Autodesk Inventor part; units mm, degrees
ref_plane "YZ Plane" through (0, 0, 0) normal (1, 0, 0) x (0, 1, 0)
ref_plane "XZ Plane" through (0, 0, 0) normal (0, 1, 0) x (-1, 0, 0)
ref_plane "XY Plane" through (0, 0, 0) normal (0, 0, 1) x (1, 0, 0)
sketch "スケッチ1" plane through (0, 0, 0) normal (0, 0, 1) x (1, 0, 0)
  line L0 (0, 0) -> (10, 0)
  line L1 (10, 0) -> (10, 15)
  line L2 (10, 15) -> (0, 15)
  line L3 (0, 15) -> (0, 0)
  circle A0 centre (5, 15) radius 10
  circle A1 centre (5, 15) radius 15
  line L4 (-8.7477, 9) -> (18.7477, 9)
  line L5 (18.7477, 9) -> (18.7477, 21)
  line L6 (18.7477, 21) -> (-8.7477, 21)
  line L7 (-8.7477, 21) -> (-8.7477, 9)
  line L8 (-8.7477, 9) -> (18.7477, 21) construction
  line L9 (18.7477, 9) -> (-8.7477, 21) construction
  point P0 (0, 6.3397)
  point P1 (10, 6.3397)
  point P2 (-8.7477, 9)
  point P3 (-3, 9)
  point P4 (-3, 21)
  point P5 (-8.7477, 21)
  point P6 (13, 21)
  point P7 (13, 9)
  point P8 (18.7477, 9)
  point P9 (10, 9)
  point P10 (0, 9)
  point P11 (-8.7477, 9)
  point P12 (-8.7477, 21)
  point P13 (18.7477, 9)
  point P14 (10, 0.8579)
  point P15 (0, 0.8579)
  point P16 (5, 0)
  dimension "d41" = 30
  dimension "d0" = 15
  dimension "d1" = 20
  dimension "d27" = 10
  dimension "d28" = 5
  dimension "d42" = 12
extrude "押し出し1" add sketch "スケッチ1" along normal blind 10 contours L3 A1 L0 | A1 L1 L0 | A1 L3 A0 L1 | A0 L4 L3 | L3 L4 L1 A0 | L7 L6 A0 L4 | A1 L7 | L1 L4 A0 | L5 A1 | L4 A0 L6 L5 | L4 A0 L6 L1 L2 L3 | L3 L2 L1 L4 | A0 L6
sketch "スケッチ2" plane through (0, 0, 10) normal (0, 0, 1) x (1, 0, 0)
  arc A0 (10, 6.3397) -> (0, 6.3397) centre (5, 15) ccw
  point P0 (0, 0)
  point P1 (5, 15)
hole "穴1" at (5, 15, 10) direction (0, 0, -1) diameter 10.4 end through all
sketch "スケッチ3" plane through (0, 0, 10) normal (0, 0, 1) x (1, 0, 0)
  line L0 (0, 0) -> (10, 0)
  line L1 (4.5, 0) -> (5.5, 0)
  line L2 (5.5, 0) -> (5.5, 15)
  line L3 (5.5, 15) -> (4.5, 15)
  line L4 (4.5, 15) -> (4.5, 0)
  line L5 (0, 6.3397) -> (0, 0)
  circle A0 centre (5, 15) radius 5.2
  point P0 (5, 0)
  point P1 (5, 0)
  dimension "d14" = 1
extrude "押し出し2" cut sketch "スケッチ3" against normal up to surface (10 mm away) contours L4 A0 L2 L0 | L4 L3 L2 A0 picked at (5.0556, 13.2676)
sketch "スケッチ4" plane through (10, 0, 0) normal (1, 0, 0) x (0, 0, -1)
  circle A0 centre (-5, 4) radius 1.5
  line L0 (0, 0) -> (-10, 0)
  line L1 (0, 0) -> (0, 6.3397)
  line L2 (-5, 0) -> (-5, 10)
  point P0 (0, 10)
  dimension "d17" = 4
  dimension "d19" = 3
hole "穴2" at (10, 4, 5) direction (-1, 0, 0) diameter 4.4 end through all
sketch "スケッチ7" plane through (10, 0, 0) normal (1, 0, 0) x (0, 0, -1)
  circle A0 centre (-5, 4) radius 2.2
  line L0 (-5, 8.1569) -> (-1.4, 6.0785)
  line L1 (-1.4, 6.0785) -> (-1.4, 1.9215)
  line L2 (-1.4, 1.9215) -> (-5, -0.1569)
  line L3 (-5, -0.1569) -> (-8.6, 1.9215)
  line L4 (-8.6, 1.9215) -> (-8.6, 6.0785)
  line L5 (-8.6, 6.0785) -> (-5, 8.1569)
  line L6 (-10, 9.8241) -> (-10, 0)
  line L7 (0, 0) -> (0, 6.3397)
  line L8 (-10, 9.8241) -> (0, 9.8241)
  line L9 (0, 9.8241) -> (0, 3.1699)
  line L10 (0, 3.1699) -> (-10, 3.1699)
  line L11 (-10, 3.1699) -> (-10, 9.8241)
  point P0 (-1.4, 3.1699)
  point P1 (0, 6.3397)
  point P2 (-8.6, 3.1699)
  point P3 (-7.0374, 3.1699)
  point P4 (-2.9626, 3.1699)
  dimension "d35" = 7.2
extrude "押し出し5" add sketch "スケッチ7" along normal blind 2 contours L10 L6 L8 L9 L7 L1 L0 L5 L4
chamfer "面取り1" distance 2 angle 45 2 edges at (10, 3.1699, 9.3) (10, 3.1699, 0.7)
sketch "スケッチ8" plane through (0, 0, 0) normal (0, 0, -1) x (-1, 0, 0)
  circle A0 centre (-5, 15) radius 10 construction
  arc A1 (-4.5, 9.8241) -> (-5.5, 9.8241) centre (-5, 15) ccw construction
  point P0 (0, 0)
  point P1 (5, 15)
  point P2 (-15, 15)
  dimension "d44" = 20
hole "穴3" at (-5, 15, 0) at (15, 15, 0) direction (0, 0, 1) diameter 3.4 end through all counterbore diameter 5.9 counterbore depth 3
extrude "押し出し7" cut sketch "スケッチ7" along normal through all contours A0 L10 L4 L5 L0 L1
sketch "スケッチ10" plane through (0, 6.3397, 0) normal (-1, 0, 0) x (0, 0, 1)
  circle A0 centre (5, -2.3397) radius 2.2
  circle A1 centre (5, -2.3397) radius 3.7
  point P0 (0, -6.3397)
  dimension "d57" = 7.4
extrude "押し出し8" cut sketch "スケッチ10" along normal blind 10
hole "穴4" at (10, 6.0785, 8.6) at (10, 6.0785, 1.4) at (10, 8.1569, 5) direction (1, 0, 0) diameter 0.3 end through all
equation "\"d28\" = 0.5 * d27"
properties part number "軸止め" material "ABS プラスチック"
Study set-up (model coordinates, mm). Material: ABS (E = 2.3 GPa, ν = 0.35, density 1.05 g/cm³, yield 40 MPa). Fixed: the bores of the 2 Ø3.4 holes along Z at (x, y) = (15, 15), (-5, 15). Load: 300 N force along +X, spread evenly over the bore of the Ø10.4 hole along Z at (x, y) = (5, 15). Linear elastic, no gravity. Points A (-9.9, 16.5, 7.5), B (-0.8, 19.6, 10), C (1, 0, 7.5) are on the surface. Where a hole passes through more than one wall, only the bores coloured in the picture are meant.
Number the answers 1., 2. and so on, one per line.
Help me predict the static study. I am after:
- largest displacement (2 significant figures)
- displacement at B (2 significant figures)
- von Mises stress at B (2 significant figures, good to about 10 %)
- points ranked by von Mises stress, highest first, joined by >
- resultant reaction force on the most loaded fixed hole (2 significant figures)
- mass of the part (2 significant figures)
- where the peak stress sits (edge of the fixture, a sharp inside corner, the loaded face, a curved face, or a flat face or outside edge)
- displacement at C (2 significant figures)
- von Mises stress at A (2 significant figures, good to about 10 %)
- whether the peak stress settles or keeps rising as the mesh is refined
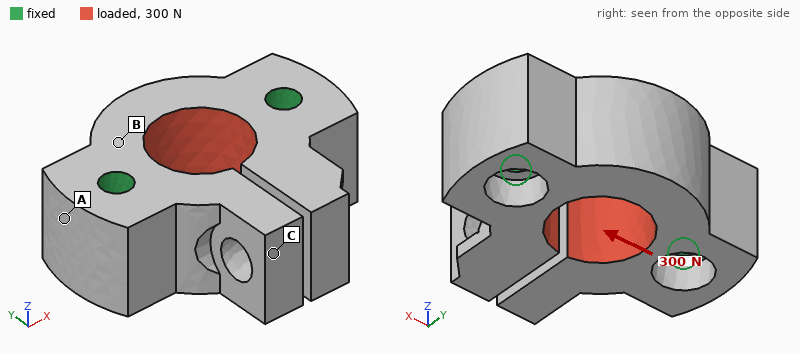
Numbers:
1. 14 µm
2. 5.7 µm
3. 1.9 MPa
4. B > A > C
5. 150 N
6. 3.8 g
7. edge of the fixture
8. 7.6 µm
9. 1.0 MPa
10. keeps rising
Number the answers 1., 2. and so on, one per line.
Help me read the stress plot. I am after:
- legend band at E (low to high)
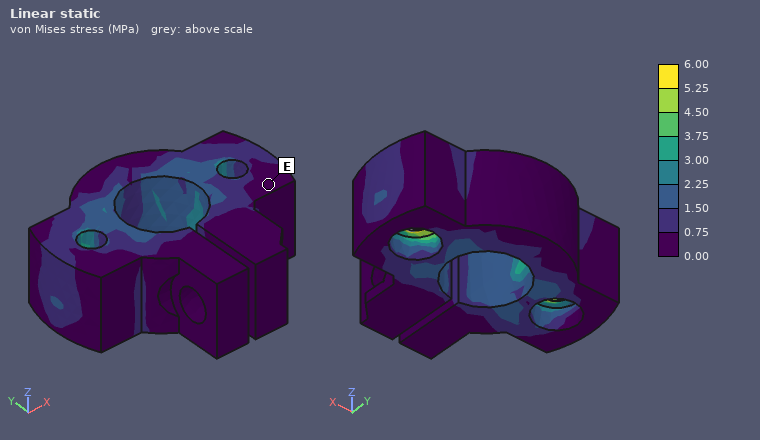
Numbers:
1. 0.00 to 0.75 MPa
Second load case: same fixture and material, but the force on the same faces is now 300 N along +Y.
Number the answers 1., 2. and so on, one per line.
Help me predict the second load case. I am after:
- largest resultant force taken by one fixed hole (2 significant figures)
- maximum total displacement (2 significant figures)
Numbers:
1. 170 N
2. 93 µm
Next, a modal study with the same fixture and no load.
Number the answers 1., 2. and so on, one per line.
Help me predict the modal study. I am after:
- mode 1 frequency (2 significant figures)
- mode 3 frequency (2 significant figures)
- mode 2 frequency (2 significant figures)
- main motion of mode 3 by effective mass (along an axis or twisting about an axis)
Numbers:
1. 5300 Hz
2. 6300 Hz
3. 5300 Hz
4. along Z
